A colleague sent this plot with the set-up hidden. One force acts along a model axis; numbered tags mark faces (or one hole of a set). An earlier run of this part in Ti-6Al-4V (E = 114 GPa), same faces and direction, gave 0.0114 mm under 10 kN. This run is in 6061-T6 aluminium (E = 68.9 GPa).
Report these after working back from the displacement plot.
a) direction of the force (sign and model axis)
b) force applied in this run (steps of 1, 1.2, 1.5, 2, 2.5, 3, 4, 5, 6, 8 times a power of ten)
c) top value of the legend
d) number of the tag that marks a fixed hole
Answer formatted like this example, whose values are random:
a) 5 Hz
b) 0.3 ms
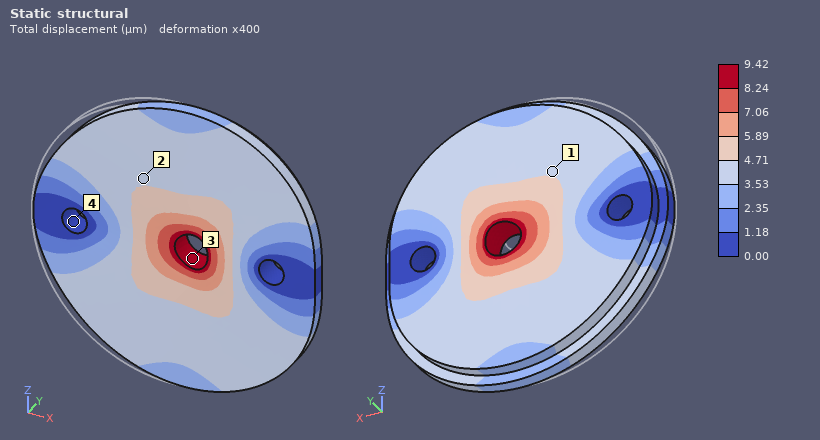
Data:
a) +X
b) 5 kN
c) 9.42 µm
d) 4
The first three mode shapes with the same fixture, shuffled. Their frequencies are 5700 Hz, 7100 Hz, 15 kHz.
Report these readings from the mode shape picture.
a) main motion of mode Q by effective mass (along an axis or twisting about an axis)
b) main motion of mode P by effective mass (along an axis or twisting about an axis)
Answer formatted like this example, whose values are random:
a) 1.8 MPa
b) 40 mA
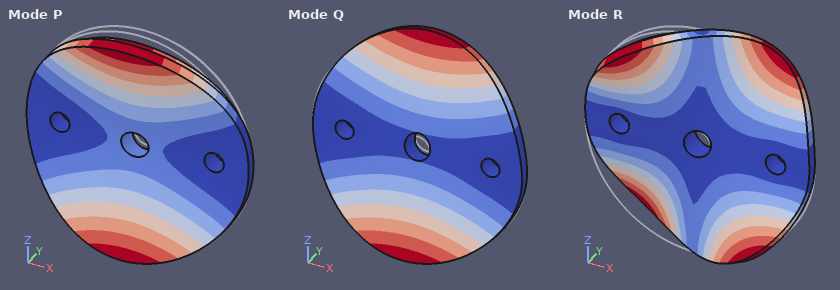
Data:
a) twisting about X
b) along Y
